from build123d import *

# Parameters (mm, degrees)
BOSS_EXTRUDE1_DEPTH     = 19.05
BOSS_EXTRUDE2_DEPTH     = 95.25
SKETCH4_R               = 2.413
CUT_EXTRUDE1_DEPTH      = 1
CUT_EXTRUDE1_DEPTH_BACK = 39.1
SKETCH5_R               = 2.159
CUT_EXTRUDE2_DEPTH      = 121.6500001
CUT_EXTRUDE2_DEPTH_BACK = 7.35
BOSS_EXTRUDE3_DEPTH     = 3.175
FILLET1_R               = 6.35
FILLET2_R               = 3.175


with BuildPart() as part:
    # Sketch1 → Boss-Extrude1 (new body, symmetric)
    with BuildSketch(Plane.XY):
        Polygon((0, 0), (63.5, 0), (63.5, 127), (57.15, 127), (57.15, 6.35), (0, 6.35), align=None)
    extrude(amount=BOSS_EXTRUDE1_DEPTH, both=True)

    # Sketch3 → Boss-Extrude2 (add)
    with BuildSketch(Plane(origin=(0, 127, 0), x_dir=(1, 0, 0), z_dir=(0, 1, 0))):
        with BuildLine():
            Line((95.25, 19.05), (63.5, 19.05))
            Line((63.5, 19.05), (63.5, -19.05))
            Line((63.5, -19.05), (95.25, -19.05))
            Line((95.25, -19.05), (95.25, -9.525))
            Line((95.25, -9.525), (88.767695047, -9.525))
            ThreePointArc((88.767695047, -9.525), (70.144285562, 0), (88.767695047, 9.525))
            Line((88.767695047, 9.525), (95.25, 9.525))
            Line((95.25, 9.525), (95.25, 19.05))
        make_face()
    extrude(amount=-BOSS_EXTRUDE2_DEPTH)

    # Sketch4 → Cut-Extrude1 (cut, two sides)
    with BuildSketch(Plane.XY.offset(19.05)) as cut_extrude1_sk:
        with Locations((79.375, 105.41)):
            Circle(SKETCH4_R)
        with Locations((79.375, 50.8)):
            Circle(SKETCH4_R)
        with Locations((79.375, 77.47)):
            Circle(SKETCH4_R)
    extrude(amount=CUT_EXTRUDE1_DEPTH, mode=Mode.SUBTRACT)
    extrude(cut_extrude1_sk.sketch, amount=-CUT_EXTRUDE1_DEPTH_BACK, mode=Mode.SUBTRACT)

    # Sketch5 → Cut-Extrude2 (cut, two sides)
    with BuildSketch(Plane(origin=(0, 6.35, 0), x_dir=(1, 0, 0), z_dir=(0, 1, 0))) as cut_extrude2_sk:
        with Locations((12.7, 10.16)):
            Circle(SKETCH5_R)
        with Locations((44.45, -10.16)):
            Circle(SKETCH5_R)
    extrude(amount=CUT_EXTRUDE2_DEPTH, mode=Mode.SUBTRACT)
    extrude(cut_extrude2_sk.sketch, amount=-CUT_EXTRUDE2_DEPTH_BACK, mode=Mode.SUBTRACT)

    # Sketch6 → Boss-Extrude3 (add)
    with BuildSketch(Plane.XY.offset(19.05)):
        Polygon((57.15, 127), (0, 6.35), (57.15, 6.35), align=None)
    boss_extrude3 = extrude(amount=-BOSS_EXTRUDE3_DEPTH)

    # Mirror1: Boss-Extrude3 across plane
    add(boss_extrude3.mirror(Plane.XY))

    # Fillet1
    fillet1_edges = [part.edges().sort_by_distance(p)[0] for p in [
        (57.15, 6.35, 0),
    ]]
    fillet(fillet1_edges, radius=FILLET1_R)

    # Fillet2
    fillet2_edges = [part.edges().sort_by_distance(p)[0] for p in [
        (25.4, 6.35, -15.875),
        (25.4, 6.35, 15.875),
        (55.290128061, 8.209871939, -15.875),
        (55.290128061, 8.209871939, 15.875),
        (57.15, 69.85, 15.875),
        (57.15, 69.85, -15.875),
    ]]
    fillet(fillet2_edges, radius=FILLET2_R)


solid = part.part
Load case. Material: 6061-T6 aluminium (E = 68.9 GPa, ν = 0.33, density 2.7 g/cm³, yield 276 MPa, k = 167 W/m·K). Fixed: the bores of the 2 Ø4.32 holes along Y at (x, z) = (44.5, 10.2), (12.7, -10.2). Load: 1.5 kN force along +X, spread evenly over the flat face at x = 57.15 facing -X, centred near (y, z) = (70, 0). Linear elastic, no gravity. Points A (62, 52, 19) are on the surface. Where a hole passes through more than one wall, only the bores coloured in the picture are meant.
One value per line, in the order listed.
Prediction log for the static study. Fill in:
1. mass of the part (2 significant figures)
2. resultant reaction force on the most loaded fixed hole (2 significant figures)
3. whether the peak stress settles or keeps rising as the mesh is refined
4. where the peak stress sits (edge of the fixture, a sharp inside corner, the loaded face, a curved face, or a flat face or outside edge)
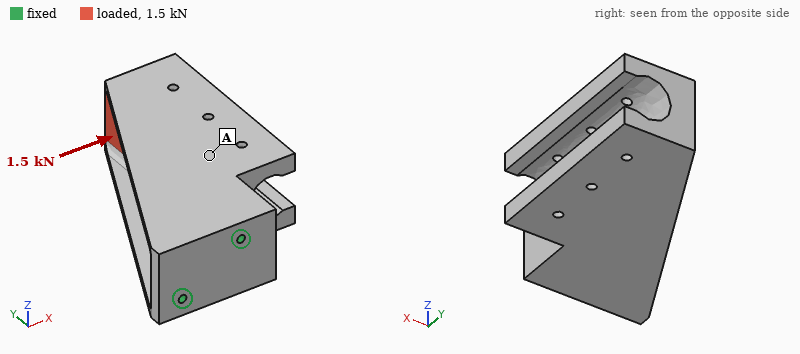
360 g
2.0 kN
keeps rising
edge of the fixture
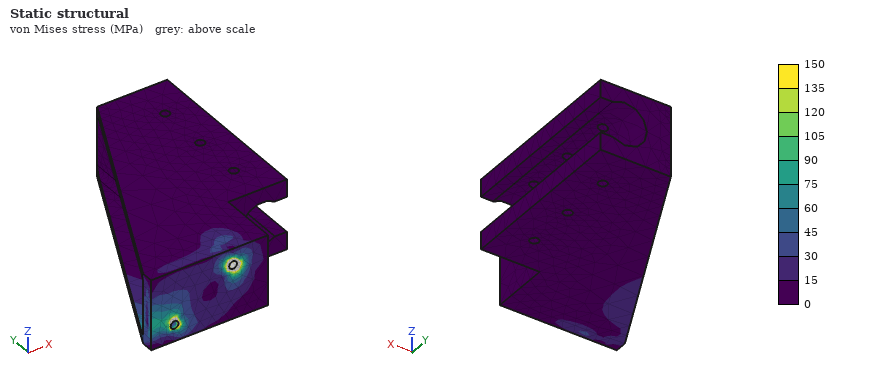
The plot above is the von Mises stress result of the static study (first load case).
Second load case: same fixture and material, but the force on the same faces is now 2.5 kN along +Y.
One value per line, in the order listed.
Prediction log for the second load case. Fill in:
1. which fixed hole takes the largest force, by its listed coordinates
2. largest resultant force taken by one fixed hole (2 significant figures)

(44.5, 10.2)
2.5 kN
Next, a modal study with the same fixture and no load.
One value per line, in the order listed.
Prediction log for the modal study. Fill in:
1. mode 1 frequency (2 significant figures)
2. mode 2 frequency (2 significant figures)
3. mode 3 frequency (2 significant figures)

400 Hz
890 Hz
2000 Hz
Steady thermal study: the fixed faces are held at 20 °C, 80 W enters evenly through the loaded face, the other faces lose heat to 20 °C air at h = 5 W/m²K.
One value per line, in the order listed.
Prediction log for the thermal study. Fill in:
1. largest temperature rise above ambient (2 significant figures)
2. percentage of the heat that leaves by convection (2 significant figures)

60 K
9.7 %
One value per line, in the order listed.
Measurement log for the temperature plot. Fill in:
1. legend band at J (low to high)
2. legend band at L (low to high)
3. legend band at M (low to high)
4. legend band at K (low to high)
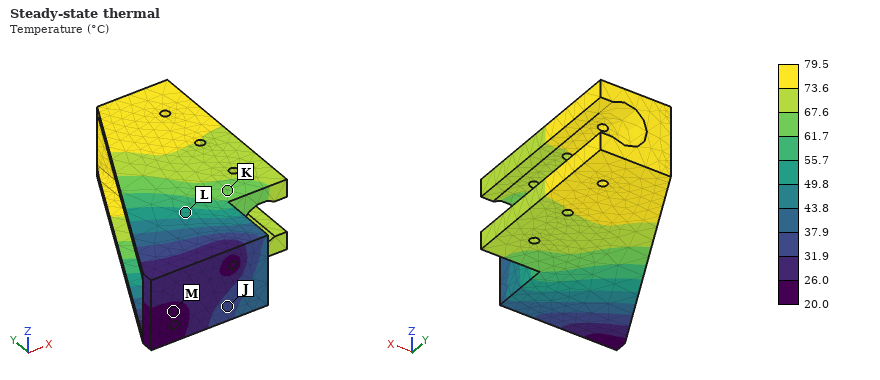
31.9 to 37.9 °C
49.8 to 55.7 °C
20.0 to 26.0 °C
61.7 to 67.6 °C
